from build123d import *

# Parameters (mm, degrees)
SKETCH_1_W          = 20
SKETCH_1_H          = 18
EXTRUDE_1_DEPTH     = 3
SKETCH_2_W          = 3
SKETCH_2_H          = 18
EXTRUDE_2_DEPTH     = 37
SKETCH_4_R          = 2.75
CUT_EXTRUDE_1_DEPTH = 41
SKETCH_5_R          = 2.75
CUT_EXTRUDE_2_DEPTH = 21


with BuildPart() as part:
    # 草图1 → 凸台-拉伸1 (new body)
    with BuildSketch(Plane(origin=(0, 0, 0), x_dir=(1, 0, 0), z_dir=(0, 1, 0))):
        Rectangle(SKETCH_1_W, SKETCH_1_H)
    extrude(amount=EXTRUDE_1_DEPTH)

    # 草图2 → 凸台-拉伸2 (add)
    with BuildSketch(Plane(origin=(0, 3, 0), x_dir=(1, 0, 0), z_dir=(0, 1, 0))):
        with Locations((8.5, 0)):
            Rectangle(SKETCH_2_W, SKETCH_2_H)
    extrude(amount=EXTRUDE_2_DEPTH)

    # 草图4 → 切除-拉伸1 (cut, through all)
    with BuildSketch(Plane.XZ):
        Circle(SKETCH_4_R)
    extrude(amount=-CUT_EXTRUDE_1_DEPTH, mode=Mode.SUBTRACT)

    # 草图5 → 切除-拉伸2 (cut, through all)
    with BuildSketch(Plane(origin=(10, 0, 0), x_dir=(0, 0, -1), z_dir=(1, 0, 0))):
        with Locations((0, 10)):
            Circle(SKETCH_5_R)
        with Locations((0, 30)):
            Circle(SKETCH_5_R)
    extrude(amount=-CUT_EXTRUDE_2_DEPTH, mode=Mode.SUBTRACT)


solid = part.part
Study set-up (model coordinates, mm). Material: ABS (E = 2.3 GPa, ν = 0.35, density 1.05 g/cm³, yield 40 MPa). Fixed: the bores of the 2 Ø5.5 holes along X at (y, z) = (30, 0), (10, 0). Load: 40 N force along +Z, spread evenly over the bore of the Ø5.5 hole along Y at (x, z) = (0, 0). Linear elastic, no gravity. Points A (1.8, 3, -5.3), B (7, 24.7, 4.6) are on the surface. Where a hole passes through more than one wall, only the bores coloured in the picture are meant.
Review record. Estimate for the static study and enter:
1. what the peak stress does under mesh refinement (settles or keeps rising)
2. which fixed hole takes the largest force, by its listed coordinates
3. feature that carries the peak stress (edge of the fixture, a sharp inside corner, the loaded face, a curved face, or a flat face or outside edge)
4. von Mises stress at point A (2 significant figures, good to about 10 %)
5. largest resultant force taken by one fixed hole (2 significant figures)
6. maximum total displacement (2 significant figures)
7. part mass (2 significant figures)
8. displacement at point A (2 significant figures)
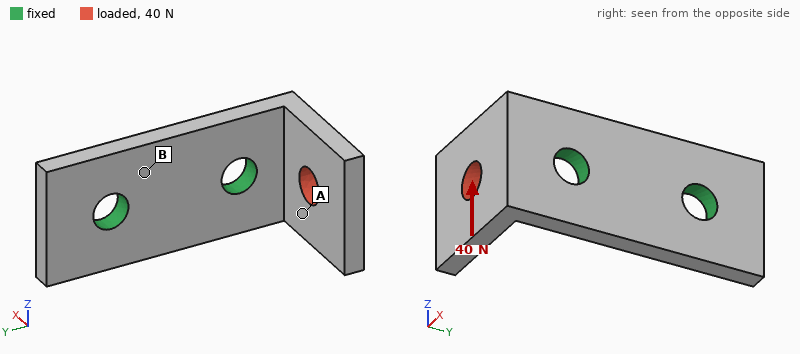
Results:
keeps rising
(10, 0)
edge of the fixture
3.0 MPa
48 N
0.27 mm
3.0 g
0.12 mm
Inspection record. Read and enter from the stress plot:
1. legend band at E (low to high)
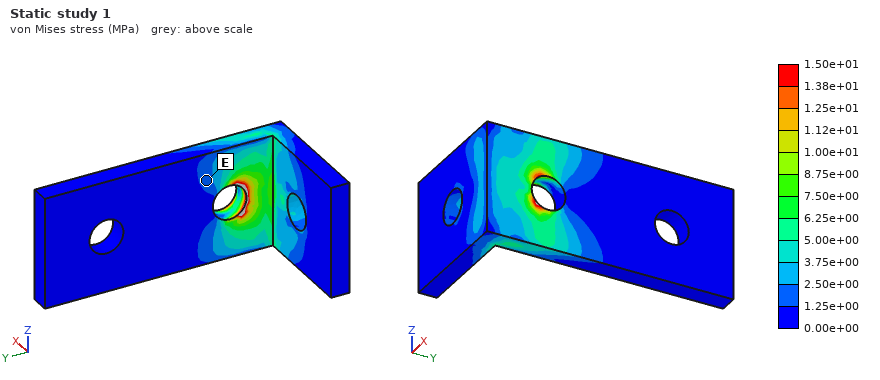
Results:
1.25e+00 to 2.50e+00 MPa
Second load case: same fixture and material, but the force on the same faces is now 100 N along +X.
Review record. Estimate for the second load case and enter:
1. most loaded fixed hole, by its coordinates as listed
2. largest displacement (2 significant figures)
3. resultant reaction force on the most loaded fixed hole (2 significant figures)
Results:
(10, 0)
0.53 mm
100 N
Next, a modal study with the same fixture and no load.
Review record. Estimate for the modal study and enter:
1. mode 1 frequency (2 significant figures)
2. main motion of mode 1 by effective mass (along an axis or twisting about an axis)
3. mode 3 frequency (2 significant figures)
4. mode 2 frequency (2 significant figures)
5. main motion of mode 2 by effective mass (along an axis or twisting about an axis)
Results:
1400 Hz
along Y
4200 Hz
2100 Hz
along Z
